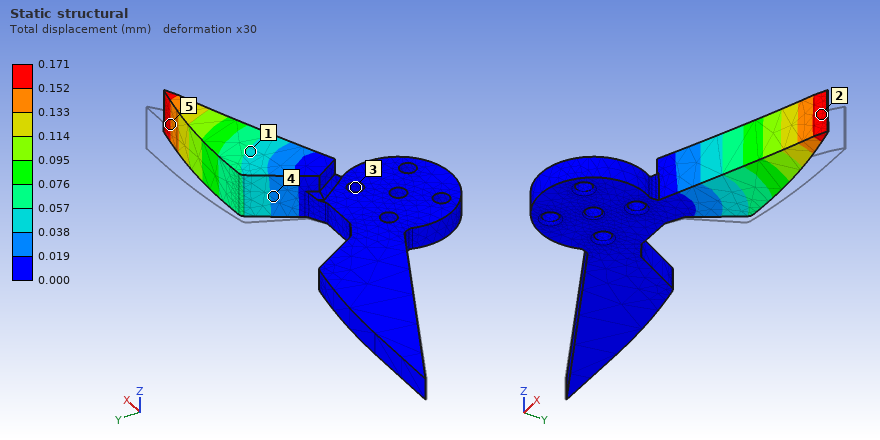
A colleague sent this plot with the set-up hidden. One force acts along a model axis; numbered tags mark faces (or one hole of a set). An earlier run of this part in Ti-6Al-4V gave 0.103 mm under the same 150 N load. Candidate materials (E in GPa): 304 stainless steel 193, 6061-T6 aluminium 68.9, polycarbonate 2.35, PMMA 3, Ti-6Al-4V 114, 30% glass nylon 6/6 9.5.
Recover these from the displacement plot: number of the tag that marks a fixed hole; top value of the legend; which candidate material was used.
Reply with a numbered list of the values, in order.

1. 3
2. 0.171 mm
3. 6061-T6 aluminium
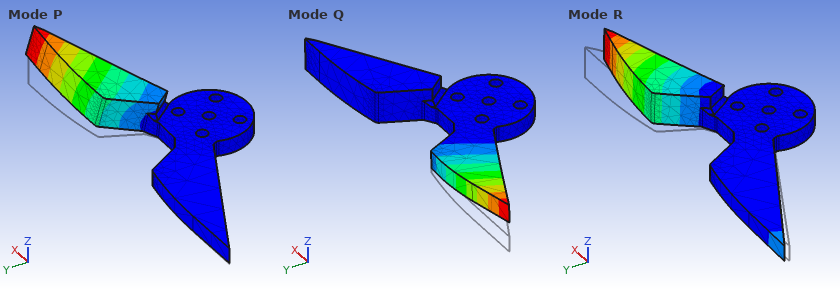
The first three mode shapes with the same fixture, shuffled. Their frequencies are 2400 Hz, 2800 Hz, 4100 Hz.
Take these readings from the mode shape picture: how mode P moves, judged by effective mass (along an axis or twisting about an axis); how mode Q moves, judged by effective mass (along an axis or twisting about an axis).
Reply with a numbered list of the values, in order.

1. along Z
2. along Z
